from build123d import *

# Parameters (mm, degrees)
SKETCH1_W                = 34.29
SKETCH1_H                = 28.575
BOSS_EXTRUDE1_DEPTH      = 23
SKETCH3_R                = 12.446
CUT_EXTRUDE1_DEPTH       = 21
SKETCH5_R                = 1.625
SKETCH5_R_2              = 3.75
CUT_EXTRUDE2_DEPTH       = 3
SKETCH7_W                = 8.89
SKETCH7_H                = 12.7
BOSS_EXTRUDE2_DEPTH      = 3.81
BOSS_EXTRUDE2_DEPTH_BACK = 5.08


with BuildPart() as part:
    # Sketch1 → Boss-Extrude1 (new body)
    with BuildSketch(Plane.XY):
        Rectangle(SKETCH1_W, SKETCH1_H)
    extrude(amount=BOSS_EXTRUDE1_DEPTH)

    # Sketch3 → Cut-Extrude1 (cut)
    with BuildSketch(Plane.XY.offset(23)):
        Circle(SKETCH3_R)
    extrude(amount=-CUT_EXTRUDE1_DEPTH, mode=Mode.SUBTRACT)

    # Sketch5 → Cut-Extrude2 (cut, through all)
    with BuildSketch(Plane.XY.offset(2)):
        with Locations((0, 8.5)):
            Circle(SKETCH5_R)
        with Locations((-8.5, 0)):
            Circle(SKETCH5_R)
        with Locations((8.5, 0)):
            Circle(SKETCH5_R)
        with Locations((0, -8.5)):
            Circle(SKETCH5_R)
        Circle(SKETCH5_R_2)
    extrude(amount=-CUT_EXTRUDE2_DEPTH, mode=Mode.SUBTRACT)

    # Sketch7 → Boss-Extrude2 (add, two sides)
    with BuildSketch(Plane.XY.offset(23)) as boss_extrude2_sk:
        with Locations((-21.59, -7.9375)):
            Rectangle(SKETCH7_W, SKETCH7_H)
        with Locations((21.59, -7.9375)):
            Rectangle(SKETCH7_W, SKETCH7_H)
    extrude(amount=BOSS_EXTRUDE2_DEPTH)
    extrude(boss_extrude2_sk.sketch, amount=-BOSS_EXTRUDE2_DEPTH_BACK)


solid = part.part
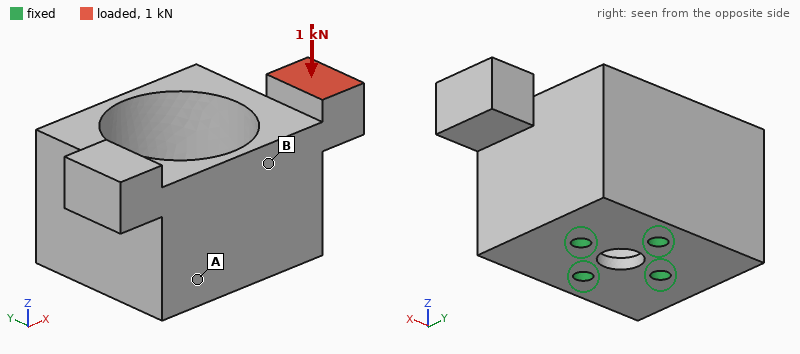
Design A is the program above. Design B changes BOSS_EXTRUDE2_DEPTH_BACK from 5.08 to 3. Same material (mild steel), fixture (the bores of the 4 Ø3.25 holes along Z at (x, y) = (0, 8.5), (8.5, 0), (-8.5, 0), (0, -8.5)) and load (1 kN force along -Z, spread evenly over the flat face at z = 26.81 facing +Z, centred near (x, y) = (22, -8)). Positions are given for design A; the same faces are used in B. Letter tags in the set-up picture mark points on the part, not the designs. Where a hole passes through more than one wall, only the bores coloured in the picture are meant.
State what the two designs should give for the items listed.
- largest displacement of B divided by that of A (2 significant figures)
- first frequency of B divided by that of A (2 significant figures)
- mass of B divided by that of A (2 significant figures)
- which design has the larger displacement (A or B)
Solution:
1.4
1.0
0.97
B
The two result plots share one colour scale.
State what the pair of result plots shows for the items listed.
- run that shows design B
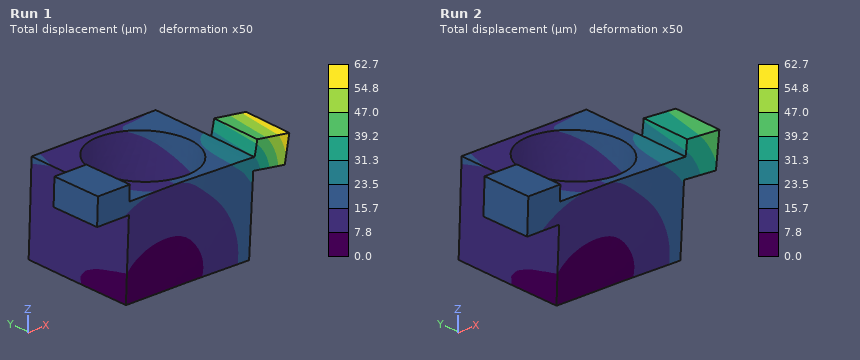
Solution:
Run 1
